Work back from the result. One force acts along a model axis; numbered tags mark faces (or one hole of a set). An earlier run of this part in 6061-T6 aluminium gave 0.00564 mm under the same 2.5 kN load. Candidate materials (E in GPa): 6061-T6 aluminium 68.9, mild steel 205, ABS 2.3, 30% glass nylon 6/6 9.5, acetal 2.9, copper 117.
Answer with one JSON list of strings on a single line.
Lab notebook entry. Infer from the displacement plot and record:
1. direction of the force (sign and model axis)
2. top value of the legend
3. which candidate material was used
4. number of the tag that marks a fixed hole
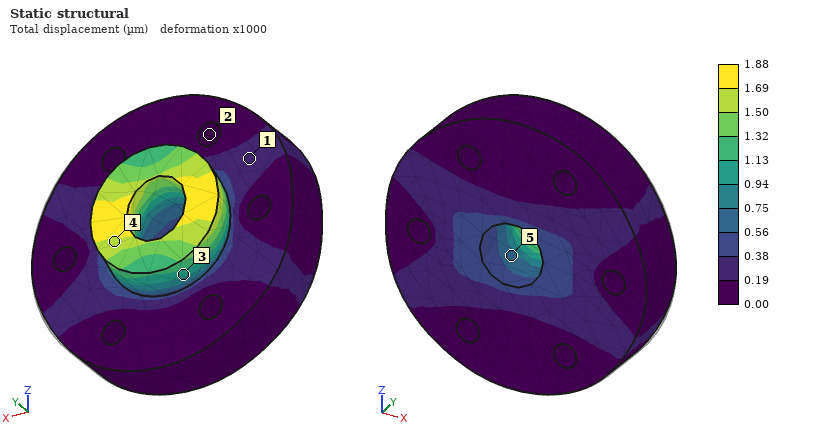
["-X", "1.88 µm", "mild steel", "2"]
